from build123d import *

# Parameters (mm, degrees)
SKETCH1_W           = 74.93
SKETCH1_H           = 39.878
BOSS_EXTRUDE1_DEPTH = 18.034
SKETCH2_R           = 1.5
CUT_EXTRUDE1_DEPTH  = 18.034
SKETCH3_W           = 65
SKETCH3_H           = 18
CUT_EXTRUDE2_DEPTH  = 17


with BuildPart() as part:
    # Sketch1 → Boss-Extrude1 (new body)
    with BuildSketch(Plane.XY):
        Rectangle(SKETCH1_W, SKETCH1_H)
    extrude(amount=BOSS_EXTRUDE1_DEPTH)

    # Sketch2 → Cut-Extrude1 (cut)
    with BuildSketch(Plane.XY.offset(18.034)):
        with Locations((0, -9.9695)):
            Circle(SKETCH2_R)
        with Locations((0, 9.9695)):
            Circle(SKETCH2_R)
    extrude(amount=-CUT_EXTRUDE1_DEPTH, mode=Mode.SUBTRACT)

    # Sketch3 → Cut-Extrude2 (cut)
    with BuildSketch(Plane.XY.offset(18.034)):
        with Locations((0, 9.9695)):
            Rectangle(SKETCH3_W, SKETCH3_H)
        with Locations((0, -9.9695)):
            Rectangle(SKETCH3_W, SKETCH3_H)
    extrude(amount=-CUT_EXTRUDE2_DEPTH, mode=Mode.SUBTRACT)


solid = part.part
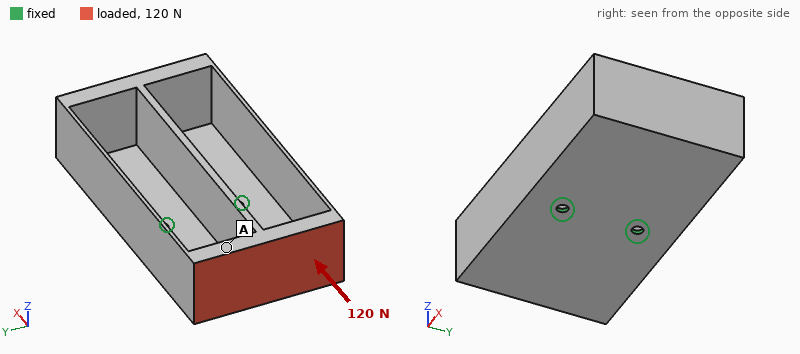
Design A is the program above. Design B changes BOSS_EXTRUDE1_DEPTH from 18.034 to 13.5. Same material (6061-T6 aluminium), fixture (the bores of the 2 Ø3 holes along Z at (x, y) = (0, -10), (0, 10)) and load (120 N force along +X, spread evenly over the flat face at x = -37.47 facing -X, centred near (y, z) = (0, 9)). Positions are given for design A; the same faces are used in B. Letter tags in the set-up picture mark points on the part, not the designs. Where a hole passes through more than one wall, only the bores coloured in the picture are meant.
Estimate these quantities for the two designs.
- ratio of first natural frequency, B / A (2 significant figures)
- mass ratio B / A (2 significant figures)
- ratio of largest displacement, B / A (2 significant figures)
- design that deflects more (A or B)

1.2
0.79
0.71
A
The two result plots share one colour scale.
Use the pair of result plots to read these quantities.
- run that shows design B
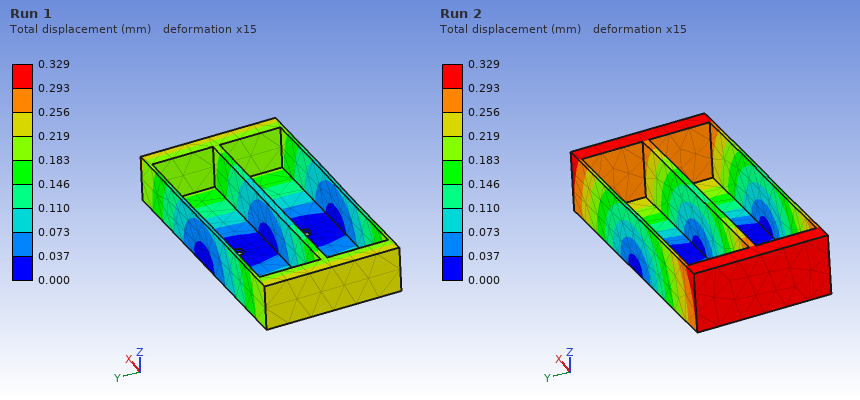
Run 1
